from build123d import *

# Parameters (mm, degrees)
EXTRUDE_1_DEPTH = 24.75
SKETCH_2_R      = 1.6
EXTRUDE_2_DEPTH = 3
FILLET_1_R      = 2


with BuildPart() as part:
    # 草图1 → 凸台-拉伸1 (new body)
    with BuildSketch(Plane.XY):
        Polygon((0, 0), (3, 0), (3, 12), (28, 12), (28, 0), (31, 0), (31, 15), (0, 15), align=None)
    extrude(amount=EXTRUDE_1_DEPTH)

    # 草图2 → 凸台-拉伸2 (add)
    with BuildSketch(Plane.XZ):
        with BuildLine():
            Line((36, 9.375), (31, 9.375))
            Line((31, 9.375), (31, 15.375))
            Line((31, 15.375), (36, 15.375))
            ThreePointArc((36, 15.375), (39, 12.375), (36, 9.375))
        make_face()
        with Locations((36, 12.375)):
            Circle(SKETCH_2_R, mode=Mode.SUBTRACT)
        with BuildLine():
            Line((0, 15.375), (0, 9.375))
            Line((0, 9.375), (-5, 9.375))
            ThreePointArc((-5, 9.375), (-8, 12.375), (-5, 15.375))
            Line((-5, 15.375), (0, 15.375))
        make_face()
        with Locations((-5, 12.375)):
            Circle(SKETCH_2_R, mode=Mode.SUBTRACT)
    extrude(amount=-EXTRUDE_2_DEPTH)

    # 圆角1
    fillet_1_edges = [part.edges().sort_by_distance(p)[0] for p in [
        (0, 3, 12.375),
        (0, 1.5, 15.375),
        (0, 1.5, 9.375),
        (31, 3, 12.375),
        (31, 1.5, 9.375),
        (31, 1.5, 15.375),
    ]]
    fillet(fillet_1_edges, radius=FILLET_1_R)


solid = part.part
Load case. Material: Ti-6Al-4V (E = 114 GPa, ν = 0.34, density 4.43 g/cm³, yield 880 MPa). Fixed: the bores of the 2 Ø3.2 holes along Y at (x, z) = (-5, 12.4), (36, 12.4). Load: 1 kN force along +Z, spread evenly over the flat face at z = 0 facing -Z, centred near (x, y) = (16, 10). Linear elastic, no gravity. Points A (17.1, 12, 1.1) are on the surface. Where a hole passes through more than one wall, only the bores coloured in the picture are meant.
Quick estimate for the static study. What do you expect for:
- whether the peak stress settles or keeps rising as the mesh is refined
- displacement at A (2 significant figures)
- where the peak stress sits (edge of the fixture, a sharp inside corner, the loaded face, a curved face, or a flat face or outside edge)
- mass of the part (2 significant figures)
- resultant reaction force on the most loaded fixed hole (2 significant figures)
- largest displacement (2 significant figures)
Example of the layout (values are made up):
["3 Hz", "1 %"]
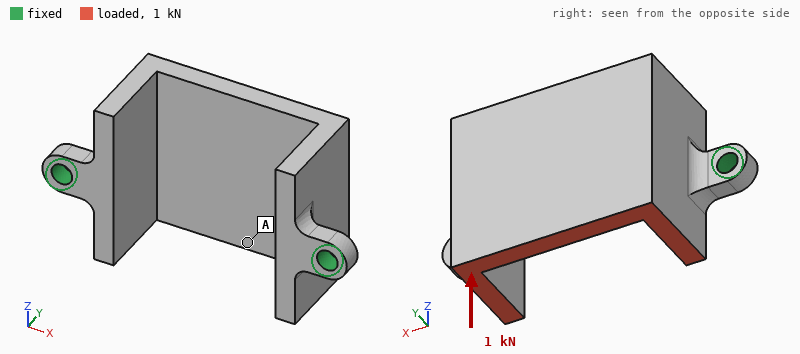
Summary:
["keeps rising", "0.15 mm", "edge of the fixture", "19 g", "500 N", "0.17 mm"]
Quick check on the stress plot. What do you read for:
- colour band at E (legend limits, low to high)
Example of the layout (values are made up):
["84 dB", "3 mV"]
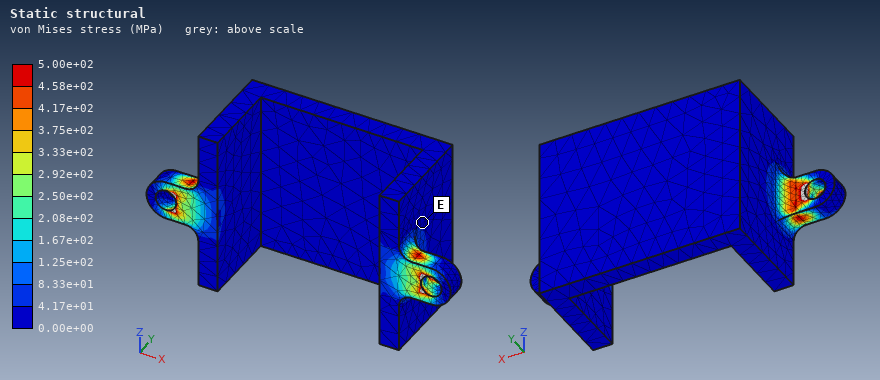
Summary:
["0.00e+00 to 4.17e+01 MPa"]
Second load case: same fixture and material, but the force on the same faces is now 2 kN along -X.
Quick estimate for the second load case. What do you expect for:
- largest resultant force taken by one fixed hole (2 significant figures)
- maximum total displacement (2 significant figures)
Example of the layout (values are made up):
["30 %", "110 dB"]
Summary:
["1.2 kN", "0.16 mm"]
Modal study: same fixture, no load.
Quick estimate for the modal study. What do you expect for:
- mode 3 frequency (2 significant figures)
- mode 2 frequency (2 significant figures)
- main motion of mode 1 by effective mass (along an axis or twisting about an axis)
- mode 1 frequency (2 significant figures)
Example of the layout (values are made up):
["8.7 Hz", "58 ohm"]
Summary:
["7000 Hz", "6800 Hz", "along Z", "3000 Hz"]
